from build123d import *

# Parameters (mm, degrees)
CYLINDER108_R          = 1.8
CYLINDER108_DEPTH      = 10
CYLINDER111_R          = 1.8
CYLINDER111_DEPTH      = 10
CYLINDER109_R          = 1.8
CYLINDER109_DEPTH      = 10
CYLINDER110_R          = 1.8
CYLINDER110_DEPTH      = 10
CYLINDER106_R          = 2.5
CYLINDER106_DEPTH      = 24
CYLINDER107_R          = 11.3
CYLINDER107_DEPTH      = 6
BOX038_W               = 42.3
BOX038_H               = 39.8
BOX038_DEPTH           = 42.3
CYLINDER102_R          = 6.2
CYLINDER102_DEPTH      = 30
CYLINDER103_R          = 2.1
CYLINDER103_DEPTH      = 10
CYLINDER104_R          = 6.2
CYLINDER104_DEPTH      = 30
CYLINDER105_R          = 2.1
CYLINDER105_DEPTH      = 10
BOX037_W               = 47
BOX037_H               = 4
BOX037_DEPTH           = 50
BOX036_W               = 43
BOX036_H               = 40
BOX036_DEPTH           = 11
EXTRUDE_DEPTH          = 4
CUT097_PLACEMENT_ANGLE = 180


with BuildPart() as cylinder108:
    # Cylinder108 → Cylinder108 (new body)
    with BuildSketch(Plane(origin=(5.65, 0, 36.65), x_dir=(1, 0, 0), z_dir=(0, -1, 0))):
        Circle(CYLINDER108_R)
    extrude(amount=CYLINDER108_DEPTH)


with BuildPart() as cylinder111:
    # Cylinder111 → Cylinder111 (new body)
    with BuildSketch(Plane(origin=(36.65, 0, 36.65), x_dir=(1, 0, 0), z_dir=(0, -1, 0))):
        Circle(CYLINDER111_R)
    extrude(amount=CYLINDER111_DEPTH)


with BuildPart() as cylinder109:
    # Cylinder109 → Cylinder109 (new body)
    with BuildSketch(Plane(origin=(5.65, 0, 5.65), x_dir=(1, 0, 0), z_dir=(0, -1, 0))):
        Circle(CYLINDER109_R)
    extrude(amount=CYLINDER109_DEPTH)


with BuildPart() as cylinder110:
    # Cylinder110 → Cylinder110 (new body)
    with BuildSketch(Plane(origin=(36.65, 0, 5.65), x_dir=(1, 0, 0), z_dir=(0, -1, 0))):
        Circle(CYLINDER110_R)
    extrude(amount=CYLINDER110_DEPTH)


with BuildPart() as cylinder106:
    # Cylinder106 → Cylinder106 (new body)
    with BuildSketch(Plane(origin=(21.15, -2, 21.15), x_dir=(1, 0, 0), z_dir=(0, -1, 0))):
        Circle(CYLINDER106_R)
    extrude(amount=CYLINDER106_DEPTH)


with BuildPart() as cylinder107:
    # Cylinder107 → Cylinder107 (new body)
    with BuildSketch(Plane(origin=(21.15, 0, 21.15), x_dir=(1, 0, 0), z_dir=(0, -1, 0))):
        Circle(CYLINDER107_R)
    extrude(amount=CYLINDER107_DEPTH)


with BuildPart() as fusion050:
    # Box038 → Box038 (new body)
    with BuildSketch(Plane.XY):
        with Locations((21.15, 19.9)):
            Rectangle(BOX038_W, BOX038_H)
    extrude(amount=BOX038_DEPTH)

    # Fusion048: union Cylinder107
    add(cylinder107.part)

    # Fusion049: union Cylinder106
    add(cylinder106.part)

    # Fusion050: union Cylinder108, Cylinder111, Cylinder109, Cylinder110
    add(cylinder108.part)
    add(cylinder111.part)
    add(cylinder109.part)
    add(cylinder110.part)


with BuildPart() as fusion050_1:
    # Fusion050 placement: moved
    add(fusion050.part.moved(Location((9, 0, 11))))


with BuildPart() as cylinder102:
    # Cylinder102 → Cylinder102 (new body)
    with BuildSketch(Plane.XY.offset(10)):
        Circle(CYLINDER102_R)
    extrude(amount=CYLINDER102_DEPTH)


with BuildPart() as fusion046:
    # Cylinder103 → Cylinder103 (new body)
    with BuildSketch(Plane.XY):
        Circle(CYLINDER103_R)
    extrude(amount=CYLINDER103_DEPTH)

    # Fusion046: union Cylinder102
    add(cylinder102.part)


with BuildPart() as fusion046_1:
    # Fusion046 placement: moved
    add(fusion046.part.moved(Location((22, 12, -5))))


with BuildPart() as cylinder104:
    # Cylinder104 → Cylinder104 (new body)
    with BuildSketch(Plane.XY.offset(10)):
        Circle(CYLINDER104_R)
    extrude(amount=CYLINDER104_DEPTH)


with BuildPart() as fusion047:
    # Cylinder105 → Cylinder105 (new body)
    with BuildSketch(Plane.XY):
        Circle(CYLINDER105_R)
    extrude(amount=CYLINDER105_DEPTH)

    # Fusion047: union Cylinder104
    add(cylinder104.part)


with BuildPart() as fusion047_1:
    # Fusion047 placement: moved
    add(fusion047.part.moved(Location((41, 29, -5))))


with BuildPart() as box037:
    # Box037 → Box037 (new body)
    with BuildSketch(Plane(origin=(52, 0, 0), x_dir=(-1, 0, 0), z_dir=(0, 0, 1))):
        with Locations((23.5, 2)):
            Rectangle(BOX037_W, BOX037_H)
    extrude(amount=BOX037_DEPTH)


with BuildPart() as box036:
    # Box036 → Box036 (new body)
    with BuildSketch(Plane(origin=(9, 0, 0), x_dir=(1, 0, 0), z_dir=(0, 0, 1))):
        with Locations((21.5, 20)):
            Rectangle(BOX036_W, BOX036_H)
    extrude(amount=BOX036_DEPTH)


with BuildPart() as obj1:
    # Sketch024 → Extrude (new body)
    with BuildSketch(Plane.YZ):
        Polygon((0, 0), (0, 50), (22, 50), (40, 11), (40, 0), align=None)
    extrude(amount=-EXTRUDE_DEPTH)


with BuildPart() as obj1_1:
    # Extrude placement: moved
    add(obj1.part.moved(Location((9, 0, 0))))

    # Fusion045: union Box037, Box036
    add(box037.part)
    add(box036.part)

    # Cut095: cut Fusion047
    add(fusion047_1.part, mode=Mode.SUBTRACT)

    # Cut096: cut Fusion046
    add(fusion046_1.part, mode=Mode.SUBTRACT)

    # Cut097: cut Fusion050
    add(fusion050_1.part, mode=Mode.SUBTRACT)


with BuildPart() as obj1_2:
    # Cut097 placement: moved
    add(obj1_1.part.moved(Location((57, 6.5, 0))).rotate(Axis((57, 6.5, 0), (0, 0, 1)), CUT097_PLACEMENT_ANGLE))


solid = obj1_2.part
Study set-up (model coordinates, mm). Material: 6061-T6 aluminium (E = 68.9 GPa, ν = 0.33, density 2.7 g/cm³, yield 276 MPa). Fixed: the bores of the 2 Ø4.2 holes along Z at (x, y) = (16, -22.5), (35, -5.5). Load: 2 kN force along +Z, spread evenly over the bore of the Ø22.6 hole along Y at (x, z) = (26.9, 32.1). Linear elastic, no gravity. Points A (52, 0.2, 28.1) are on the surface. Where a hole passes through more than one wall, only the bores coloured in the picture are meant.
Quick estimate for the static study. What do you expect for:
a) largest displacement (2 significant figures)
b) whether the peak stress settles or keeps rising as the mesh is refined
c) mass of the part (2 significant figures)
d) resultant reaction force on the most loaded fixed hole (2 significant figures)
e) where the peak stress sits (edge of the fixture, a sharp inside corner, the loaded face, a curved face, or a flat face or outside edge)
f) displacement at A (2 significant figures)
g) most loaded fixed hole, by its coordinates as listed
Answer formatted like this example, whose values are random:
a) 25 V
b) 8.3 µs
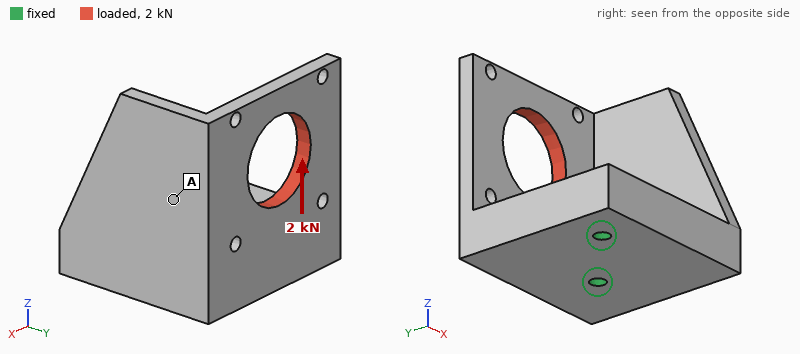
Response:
a) 0.20 mm
b) keeps rising
c) 85 g
d) 2.1 kN
e) edge of the fixture
f) 0.080 mm
g) (35, -5.5)
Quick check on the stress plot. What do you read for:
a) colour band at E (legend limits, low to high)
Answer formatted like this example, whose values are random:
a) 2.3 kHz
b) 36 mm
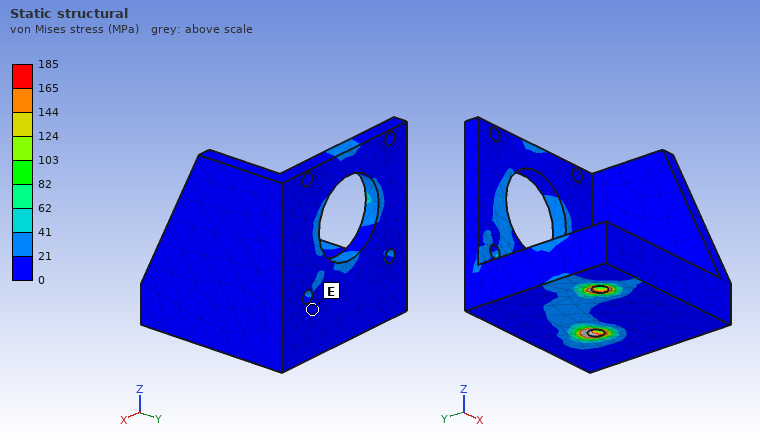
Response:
a) 0 to 21 MPa
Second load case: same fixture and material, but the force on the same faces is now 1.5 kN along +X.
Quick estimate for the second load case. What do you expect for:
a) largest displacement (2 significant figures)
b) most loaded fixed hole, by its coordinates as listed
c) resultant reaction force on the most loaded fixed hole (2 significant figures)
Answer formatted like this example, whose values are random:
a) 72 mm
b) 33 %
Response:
a) 0.24 mm
b) (35, -5.5)
c) 2.0 kN
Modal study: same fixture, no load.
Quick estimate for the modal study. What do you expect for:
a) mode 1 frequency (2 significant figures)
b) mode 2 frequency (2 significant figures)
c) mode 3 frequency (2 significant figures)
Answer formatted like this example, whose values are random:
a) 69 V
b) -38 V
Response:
a) 2200 Hz
b) 3200 Hz
c) 3900 Hz
